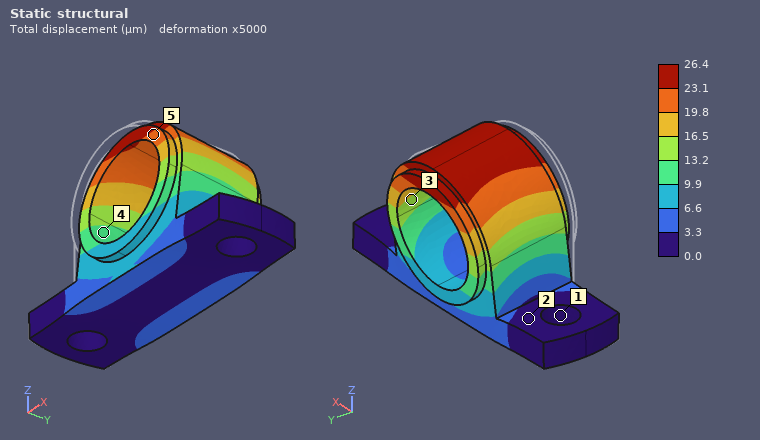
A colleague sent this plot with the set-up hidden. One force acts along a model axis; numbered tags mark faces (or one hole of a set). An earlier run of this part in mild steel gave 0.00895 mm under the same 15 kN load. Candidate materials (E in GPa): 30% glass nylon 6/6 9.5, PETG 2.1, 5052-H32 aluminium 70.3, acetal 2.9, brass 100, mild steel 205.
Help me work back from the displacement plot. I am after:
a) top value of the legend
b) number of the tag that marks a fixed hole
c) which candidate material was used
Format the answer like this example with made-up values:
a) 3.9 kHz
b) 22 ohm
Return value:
a) 26.4 µm
b) 1
c) 5052-H32 aluminium
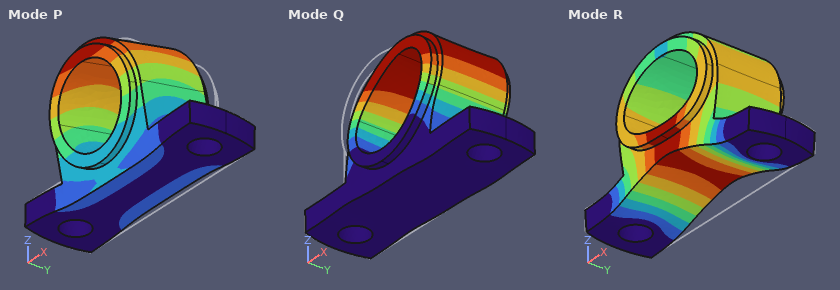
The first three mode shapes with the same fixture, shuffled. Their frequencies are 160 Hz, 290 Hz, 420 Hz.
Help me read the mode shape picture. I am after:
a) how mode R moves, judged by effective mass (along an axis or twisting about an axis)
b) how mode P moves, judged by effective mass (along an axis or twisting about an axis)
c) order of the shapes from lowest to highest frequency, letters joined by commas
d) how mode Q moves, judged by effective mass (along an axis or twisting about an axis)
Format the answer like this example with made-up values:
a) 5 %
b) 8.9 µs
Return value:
a) along Z
b) along Y
c) P, Q, R
d) along X
